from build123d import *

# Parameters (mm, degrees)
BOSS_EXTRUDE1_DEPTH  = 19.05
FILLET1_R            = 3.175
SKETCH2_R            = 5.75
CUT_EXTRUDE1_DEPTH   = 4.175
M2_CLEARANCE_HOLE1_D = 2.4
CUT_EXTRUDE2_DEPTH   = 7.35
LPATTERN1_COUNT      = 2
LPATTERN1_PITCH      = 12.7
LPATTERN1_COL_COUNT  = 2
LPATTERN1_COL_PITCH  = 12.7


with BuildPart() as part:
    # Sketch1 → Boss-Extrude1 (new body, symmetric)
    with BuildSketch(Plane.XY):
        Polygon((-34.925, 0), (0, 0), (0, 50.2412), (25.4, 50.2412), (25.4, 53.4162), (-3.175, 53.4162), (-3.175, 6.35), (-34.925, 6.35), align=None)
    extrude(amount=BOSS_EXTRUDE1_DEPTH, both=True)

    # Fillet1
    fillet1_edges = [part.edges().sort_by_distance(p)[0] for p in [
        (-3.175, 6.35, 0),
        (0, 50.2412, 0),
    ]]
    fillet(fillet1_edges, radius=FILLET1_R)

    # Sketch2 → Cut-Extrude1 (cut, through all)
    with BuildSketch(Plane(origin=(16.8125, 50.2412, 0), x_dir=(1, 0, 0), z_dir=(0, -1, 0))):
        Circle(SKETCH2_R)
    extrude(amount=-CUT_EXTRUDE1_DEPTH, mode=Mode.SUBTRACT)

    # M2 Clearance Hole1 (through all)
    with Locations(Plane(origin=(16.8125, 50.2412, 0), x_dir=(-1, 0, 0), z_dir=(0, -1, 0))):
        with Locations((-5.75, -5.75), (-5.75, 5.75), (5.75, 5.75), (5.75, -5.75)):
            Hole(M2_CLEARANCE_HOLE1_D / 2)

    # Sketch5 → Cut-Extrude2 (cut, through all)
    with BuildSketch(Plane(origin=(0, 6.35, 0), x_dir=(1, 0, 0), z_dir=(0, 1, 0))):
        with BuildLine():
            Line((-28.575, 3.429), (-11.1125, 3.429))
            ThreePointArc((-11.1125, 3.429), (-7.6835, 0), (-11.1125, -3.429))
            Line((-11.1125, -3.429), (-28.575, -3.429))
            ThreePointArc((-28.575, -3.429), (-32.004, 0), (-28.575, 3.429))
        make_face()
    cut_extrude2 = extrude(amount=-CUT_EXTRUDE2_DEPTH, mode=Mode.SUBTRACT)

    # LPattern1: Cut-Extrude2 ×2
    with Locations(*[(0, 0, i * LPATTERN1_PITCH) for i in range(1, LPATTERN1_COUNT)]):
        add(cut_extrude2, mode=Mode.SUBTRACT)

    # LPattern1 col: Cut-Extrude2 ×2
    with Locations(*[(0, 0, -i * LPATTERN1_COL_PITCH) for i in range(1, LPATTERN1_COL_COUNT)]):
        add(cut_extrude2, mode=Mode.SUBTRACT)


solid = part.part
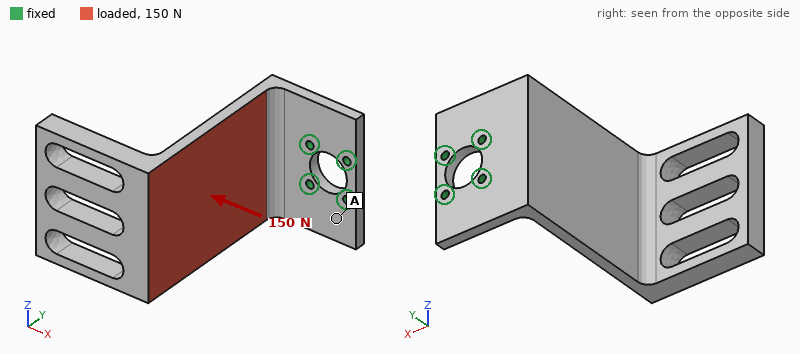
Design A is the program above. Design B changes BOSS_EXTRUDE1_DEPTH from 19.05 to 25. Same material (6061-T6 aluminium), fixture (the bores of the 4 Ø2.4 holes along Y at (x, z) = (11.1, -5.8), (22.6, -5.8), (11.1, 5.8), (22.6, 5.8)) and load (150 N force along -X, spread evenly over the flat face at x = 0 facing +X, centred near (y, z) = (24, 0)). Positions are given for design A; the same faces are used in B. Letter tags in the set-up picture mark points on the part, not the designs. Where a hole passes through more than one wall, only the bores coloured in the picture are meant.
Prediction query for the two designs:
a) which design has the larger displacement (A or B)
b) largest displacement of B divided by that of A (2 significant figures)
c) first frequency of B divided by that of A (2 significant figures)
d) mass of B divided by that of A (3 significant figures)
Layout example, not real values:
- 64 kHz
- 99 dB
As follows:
- A
- 0.79
- 0.93
- 1.39
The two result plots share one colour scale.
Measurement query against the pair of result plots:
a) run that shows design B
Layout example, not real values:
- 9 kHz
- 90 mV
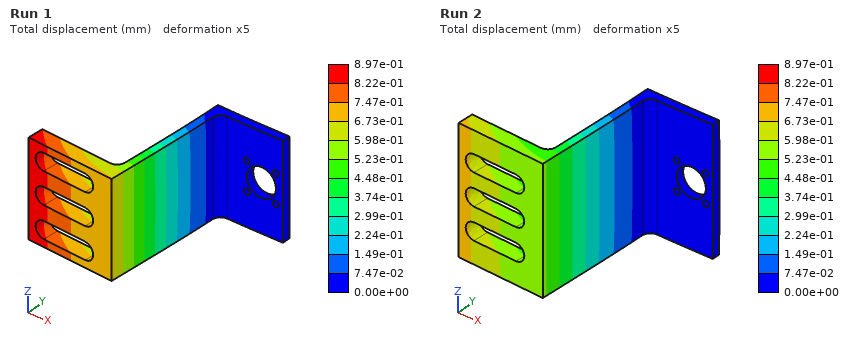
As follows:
- Run 2
